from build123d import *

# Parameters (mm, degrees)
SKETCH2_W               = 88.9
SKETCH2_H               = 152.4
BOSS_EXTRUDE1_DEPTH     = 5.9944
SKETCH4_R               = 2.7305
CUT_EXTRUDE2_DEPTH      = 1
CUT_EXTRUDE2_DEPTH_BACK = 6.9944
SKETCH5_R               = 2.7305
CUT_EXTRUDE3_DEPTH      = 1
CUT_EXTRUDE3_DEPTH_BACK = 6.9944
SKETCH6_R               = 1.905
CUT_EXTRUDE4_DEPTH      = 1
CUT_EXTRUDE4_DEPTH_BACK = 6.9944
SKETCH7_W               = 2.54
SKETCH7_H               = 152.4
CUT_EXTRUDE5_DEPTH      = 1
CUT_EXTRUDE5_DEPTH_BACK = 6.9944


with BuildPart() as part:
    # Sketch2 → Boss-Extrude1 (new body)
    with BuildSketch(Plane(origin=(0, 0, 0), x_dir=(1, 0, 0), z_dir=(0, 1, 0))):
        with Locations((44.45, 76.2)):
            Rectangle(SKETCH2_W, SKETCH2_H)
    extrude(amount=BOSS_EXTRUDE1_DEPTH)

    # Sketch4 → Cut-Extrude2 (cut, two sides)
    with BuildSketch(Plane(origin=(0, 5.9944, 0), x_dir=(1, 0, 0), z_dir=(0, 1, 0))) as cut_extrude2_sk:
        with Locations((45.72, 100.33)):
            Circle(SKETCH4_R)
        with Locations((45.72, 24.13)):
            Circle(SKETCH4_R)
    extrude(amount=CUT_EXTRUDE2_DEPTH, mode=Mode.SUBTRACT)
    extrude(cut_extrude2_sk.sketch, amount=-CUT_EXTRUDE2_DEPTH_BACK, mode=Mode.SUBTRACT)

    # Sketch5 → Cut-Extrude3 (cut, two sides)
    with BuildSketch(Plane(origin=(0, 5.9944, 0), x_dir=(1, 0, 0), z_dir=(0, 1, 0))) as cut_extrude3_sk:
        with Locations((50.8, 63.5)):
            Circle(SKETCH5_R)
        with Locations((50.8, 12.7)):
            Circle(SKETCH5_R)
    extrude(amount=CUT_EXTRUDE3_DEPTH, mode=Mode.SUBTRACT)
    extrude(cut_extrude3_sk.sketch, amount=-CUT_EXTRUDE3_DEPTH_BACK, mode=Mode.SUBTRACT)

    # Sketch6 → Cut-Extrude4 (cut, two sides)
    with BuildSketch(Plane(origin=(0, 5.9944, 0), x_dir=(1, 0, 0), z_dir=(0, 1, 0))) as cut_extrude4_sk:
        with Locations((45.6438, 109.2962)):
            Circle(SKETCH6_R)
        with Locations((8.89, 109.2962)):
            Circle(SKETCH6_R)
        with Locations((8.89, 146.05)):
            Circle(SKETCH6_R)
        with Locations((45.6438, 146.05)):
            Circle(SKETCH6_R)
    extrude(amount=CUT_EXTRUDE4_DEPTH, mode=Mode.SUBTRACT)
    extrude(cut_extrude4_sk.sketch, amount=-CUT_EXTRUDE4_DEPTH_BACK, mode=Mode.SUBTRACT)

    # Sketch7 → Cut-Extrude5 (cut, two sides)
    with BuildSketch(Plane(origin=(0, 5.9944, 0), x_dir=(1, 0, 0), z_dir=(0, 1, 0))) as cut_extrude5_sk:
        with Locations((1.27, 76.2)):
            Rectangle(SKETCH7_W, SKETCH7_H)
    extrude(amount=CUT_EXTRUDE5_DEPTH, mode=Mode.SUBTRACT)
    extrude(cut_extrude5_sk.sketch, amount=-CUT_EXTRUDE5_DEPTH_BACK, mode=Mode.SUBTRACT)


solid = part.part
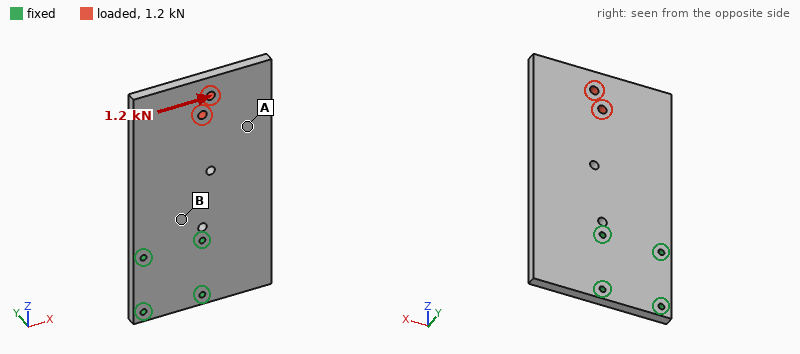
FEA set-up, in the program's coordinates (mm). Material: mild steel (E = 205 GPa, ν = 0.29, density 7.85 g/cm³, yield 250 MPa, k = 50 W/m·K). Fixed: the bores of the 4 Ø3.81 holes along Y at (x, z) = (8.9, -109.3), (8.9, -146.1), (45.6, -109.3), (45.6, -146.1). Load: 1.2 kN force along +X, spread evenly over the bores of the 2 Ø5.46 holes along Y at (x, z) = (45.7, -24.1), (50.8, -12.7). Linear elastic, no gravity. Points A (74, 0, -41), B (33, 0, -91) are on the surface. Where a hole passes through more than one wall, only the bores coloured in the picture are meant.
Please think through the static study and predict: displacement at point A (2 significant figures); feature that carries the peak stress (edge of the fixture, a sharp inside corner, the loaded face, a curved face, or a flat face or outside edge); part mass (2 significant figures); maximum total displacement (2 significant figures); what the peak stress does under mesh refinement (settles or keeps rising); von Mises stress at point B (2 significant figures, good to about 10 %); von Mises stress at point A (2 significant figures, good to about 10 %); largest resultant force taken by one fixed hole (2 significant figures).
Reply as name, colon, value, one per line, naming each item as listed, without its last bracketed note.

displacement at point A: 11 µm
feature that carries the peak stress: edge of the fixture
part mass: 610 g
maximum total displacement: 17 µm
what the peak stress does under mesh refinement: keeps rising
von Mises stress at point B: 8.8 MPa
von Mises stress at point A: 4.2 MPa
largest resultant force taken by one fixed hole: 1.9 kN
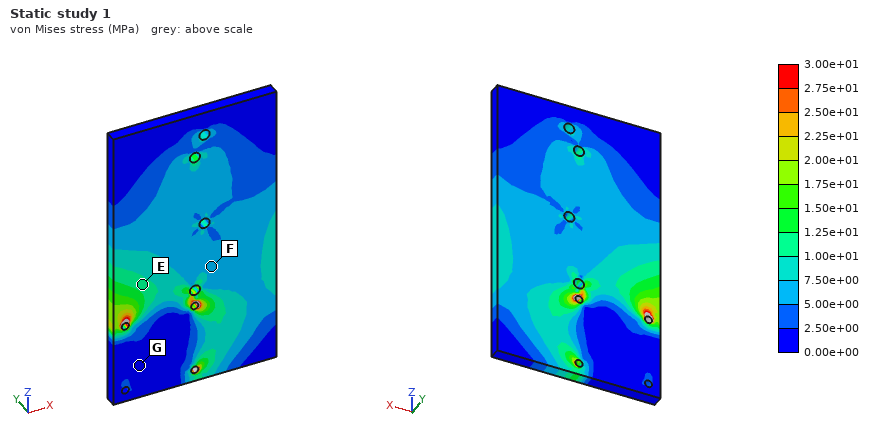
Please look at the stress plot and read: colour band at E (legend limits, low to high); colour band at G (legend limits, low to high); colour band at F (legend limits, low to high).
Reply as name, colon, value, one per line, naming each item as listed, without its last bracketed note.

colour band at E: 1.00e+01 to 1.25e+01 MPa
colour band at G: 0.00e+00 to 2.50e+00 MPa
colour band at F: 5.00e+00 to 7.50e+00 MPa
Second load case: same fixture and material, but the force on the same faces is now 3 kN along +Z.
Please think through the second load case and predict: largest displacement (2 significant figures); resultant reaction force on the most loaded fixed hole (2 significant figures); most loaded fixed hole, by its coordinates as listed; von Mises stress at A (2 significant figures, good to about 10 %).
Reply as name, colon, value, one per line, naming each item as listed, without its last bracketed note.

largest displacement: 7.1 µm
resultant reaction force on the most loaded fixed hole: 1.8 kN
most loaded fixed hole, by its coordinates as listed: (45.6, -109.3)
von Mises stress at A: 5.9 MPa
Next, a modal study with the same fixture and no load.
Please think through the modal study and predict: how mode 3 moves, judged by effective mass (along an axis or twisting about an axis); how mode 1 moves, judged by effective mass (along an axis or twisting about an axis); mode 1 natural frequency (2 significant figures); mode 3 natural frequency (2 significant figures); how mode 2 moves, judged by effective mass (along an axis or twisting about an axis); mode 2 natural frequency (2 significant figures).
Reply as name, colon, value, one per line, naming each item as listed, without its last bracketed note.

how mode 3 moves, judged by effective mass: along Y
how mode 1 moves, judged by effective mass: along Y
mode 1 natural frequency: 380 Hz
mode 3 natural frequency: 2200 Hz
how mode 2 moves, judged by effective mass: twisting about Z
mode 2 natural frequency: 1000 Hz
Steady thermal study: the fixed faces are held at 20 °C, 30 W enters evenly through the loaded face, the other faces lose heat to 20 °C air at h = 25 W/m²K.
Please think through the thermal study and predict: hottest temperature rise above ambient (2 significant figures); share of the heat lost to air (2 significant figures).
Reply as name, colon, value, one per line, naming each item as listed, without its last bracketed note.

hottest temperature rise above ambient: 82 K
share of the heat lost to air: 63 %
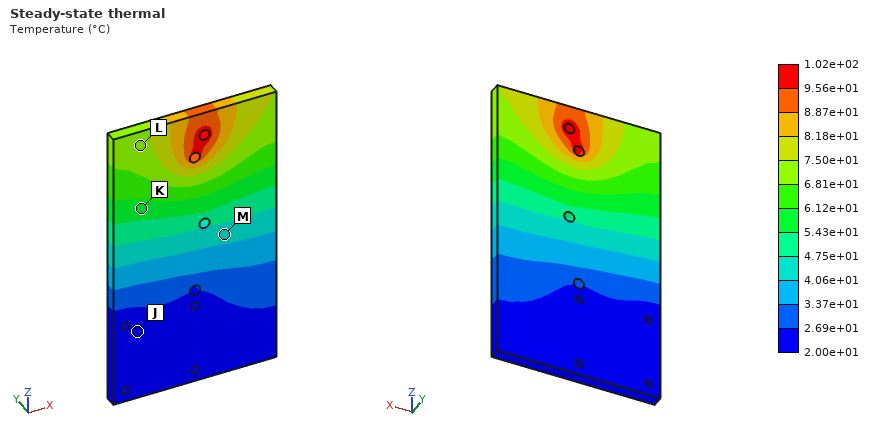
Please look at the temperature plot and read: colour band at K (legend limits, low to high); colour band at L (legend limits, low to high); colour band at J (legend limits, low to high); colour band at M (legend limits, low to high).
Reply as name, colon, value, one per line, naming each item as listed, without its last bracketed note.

colour band at K: 5.43e+01 to 6.12e+01 °C
colour band at L: 6.81e+01 to 7.50e+01 °C
colour band at J: 2.00e+01 to 2.69e+01 °C
colour band at M: 4.06e+01 to 4.75e+01 °C
